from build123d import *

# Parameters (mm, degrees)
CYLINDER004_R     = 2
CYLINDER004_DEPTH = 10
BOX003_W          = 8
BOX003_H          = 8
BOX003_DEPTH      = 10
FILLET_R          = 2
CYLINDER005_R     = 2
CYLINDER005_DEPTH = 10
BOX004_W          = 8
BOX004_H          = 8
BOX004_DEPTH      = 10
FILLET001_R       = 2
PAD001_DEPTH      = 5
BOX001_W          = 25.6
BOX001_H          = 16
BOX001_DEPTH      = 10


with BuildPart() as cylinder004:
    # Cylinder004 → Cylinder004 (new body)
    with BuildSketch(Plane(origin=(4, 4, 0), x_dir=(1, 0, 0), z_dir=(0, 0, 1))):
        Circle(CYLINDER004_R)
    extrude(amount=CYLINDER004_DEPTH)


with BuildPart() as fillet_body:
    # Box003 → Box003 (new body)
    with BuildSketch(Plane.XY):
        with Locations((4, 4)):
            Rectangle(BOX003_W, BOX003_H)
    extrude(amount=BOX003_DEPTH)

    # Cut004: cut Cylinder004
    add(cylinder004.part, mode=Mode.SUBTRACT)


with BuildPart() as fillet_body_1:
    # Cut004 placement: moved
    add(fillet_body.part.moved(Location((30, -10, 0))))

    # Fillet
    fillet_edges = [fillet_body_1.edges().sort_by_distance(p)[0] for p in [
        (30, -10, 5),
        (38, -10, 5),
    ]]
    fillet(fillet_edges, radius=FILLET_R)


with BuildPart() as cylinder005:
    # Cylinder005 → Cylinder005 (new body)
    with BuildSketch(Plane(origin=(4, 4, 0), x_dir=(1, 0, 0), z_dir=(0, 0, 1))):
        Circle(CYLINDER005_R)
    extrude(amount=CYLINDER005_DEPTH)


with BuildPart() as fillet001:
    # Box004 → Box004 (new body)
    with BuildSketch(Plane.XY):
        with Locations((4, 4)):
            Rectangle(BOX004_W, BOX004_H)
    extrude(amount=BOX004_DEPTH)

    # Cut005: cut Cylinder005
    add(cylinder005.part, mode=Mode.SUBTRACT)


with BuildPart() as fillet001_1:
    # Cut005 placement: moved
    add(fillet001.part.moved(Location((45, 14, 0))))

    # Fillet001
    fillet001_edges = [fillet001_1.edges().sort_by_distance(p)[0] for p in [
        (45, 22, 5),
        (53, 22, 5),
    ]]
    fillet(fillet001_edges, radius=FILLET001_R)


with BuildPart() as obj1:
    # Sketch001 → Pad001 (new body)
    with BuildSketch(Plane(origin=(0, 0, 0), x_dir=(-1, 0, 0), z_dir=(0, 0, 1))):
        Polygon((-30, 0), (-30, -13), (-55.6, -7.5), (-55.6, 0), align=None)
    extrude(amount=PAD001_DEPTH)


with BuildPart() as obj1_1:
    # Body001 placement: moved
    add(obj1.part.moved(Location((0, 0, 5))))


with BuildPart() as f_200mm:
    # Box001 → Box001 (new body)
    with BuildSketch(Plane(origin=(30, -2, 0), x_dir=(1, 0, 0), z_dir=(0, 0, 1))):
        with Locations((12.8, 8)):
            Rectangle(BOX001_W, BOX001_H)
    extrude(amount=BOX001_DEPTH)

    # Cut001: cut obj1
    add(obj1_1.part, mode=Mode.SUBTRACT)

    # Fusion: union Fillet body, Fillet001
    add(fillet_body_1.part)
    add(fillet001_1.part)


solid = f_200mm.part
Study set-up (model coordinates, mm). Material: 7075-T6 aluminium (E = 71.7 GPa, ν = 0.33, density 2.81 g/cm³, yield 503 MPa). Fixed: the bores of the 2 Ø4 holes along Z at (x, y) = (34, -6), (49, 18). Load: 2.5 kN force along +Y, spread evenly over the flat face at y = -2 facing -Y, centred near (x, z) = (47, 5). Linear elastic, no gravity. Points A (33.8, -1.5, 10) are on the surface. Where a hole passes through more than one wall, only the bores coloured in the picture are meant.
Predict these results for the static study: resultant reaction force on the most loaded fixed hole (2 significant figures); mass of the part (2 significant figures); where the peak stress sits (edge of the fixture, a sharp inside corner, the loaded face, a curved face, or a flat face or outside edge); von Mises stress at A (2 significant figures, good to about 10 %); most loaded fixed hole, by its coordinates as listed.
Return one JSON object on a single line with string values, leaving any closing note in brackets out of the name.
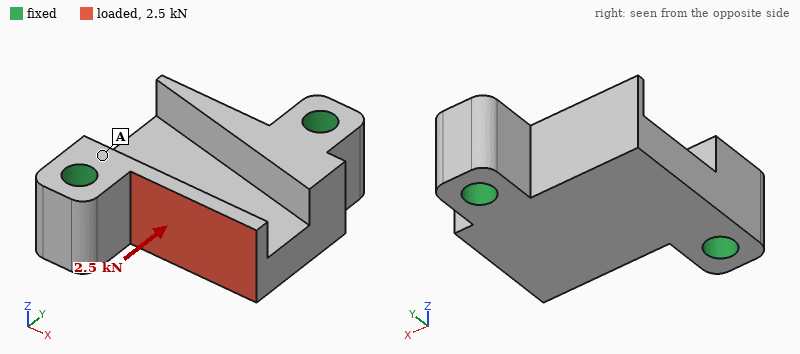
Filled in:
{"resultant reaction force on the most loaded fixed hole": "1.7 kN", "mass of the part": "11 g", "where the peak stress sits": "the loaded face", "von Mises stress at A": "29 MPa", "most loaded fixed hole, by its coordinates as listed": "(49, 18)"}
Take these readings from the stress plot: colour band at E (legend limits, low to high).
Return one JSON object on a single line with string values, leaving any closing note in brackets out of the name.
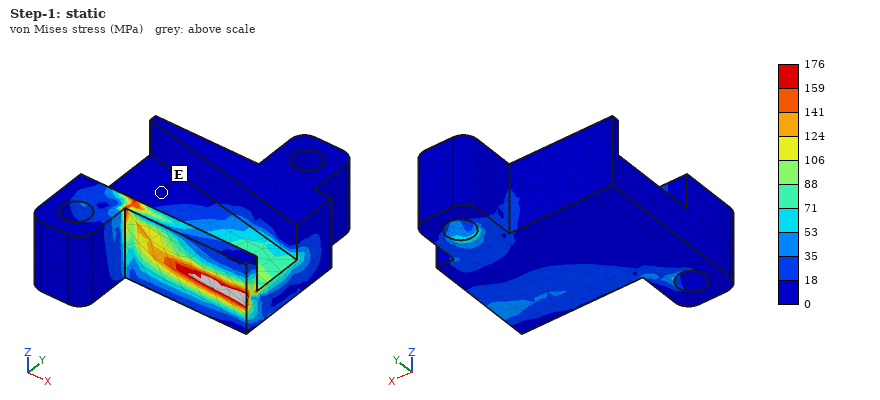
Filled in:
{"colour band at E": "0 to 18 MPa"}
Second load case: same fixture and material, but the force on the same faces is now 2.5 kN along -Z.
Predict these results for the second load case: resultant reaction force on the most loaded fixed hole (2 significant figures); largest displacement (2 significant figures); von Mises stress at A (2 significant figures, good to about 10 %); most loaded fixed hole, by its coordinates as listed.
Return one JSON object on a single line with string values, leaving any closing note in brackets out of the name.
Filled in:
{"resultant reaction force on the most loaded fixed hole": "1.7 kN", "largest displacement": "0.16 mm", "von Mises stress at A": "120 MPa", "most loaded fixed hole, by its coordinates as listed": "(34, -6)"}
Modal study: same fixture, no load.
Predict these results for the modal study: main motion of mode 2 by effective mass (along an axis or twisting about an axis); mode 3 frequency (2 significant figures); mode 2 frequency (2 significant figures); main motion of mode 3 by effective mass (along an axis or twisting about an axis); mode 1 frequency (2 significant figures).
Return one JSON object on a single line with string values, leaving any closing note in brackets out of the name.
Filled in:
{"main motion of mode 2 by effective mass": "along Z", "mode 3 frequency": "34 kHz", "mode 2 frequency": "24 kHz", "main motion of mode 3 by effective mass": "along X", "mode 1 frequency": "20 kHz"}
